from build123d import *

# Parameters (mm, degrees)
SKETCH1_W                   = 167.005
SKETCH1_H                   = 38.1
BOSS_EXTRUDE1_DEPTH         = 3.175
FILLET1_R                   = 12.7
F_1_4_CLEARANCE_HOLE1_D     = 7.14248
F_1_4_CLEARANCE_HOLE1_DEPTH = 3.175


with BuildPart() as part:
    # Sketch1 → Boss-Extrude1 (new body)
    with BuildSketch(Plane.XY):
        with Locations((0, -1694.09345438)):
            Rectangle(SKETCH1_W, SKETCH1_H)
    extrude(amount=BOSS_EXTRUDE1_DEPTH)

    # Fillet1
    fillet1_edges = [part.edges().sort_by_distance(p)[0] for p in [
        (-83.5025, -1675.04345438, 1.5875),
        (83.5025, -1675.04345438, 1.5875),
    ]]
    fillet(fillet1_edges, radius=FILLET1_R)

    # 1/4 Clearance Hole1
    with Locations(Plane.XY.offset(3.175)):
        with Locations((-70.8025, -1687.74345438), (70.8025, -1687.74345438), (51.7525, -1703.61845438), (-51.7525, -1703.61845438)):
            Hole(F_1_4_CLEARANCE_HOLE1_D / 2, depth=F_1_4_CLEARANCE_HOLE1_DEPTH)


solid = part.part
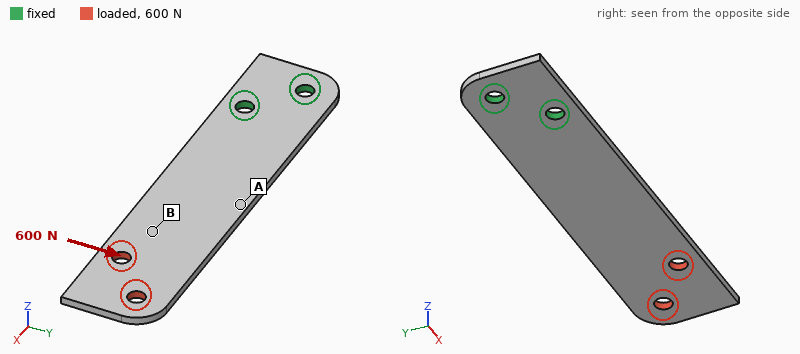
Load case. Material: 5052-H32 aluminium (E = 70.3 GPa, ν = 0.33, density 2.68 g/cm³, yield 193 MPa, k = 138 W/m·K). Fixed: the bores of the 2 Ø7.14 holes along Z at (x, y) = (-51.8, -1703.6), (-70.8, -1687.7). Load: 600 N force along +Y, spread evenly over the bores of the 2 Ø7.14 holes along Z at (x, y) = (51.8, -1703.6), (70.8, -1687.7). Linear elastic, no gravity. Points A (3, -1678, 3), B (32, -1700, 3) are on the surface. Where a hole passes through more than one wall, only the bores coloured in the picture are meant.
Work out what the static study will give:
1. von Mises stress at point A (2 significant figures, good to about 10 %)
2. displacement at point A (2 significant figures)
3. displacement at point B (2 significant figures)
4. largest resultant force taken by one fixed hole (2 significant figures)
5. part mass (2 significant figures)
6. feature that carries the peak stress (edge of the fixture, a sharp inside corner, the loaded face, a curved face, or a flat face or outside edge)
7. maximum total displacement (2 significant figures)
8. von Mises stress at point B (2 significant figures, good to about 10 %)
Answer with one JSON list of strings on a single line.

["39 MPa", "0.14 mm", "0.25 mm", "2.7 kN", "52 g", "edge of the fixture", "0.49 mm", "14 MPa"]
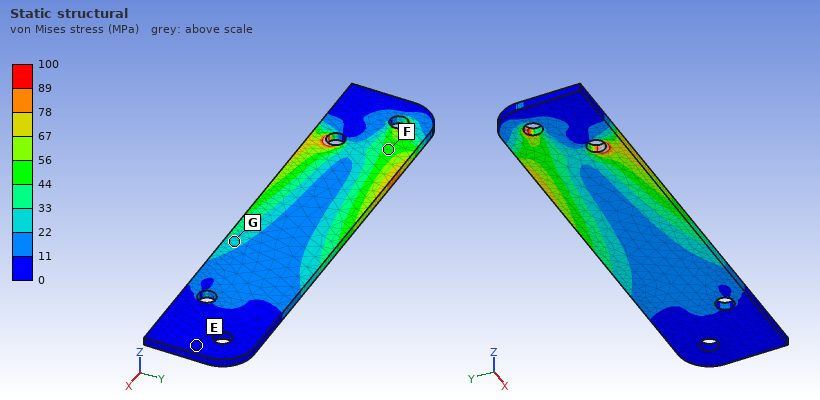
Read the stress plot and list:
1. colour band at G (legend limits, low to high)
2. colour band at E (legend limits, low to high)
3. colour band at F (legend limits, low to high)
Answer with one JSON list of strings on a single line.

["22 to 33 MPa", "0 to 11 MPa", "44 to 56 MPa"]
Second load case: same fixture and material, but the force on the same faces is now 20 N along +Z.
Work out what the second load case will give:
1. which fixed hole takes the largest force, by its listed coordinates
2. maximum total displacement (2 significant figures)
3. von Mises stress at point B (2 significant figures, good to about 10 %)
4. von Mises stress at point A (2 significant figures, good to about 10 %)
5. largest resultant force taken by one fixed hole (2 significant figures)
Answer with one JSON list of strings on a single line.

["(-51.8, -1703.6)", "1.7 mm", "9.3 MPa", "18 MPa", "60 N"]
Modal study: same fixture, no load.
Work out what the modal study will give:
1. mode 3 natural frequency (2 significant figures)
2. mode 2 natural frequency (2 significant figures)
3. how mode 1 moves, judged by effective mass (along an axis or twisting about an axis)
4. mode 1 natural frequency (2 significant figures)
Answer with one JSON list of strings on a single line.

["1000 Hz", "870 Hz", "along Z", "150 Hz"]
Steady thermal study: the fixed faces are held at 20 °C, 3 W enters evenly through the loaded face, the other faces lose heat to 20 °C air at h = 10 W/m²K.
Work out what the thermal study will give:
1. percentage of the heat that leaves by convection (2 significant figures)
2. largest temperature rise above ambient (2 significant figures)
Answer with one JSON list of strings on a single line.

["33 %", "16 K"]
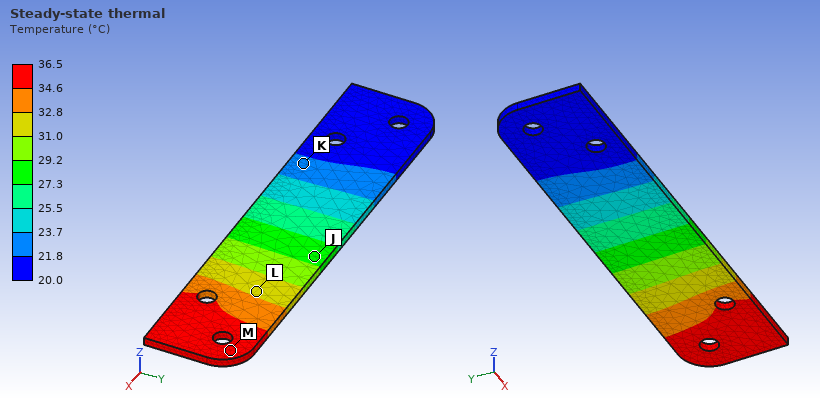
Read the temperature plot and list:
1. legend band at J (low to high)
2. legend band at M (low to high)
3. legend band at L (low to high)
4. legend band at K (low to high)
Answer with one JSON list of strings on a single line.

["27.3 to 29.2 °C", "34.6 to 36.5 °C", "31.0 to 32.8 °C", "21.8 to 23.7 °C"]
